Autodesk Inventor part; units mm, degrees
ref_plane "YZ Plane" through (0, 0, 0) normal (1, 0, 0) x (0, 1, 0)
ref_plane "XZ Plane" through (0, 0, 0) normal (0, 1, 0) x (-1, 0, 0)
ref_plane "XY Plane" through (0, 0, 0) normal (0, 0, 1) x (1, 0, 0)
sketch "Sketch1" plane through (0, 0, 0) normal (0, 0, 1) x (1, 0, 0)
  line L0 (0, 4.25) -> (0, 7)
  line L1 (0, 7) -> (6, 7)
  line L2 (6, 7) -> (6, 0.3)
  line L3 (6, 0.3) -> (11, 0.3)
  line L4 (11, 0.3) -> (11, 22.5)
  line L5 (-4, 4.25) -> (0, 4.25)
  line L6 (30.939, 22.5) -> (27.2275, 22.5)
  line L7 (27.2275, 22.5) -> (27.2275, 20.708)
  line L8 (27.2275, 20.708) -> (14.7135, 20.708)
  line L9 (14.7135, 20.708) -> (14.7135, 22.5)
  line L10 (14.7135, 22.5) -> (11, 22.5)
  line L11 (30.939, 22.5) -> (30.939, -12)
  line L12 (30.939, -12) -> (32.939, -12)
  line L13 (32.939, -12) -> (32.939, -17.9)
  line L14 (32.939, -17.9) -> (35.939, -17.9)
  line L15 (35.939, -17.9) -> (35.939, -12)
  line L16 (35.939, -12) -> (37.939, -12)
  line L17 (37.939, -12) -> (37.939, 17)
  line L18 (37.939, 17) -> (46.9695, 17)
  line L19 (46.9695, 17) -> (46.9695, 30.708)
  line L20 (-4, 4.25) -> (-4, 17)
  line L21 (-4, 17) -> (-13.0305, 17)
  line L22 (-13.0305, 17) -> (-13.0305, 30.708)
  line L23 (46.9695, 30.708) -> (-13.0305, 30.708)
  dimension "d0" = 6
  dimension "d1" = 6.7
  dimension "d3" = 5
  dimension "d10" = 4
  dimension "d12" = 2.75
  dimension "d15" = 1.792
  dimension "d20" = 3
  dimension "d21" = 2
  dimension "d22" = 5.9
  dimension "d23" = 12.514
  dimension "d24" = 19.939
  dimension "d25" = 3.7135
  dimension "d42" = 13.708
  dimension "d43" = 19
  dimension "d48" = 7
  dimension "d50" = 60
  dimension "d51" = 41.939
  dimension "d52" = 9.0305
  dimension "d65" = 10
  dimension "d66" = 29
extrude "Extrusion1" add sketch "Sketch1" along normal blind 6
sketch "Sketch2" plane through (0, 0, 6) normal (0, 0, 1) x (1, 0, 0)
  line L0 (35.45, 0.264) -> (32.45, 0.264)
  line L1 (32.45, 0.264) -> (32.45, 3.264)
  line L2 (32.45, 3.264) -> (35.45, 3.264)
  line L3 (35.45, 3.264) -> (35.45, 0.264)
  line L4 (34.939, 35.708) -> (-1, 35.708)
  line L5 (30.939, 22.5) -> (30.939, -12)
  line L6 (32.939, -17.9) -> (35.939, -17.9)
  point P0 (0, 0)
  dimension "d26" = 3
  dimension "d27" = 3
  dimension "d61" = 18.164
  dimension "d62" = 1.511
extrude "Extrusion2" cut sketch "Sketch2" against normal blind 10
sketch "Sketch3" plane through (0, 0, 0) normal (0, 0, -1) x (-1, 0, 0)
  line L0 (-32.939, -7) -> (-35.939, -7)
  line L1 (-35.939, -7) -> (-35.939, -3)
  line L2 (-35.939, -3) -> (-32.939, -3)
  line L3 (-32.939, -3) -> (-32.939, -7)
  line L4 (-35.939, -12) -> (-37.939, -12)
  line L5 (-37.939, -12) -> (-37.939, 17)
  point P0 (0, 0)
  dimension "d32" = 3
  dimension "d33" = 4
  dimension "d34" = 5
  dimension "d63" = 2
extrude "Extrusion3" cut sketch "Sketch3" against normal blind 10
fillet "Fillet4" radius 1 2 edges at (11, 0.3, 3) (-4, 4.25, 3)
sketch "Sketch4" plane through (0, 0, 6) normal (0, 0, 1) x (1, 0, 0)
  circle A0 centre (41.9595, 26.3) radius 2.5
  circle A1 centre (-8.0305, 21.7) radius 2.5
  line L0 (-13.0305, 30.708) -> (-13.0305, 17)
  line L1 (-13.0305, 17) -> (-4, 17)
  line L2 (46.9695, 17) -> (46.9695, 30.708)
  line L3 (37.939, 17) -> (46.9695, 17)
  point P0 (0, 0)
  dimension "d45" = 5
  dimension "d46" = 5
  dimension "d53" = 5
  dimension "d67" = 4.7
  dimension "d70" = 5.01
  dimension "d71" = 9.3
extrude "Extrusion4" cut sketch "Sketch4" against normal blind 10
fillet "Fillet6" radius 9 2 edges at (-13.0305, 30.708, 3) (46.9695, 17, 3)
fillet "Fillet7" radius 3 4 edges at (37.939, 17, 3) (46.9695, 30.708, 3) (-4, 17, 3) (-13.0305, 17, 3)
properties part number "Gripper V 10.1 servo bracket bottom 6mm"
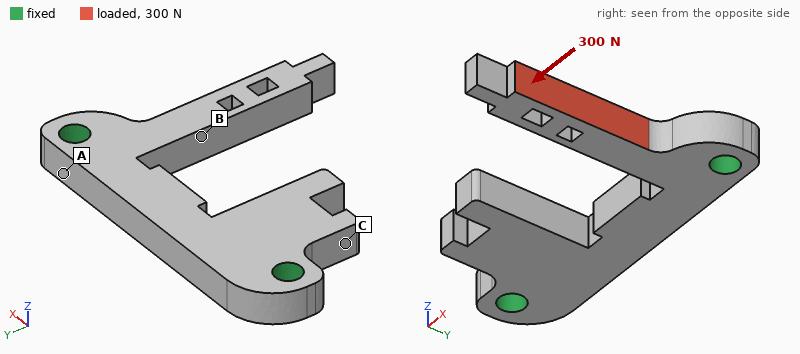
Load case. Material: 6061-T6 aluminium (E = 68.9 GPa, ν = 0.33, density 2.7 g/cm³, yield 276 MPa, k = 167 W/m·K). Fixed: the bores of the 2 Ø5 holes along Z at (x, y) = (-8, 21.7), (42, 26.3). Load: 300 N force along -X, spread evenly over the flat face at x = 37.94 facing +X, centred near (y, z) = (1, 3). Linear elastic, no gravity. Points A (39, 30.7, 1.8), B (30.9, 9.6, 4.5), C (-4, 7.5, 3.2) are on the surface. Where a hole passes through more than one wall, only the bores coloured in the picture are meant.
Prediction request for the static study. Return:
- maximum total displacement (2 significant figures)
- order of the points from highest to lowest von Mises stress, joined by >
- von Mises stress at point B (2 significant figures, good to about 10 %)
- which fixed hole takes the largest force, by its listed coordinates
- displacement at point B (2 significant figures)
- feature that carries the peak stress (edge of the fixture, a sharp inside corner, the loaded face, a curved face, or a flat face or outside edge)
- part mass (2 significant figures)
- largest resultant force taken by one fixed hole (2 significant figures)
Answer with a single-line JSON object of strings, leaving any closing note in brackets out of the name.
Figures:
{"maximum total displacement": "0.19 mm", "order of the points from highest to lowest von Mises stress, joined by >": "B > A > C", "von Mises stress at point B": "54 MPa", "which fixed hole takes the largest force, by its listed coordinates": "(42, 26.3)", "displacement at point B": "0.038 mm", "feature that carries the peak stress": "a curved face", "part mass": "17 g", "largest resultant force taken by one fixed hole": "370 N"}
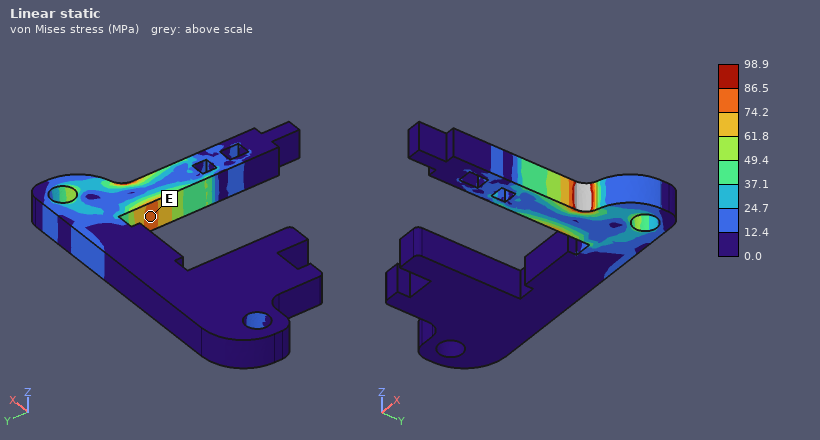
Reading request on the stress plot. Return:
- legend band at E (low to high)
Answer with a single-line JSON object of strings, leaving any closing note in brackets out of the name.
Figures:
{"legend band at E": "74.2 to 86.5 MPa"}
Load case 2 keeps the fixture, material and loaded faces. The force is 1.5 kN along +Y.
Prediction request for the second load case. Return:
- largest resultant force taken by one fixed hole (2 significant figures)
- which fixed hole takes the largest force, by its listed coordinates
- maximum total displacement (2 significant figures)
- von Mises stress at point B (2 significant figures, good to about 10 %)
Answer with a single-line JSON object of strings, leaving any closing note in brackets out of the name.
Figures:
{"largest resultant force taken by one fixed hole": "1.4 kN", "which fixed hole takes the largest force, by its listed coordinates": "(42, 26.3)", "maximum total displacement": "0.19 mm", "von Mises stress at point B": "59 MPa"}
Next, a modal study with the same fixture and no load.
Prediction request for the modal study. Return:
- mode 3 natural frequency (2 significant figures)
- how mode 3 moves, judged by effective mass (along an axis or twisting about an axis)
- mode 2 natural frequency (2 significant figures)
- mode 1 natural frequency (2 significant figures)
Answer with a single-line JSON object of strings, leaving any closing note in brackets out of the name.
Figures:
{"mode 3 natural frequency": "8700 Hz", "how mode 3 moves, judged by effective mass": "along Z", "mode 2 natural frequency": "4400 Hz", "mode 1 natural frequency": "3300 Hz"}
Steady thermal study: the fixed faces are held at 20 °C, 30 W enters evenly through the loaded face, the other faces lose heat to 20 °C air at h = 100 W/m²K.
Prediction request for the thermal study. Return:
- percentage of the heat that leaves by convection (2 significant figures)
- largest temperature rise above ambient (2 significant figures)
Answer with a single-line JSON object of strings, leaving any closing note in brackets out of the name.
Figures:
{"percentage of the heat that leaves by convection": "21 %", "largest temperature rise above ambient": "85 K"}
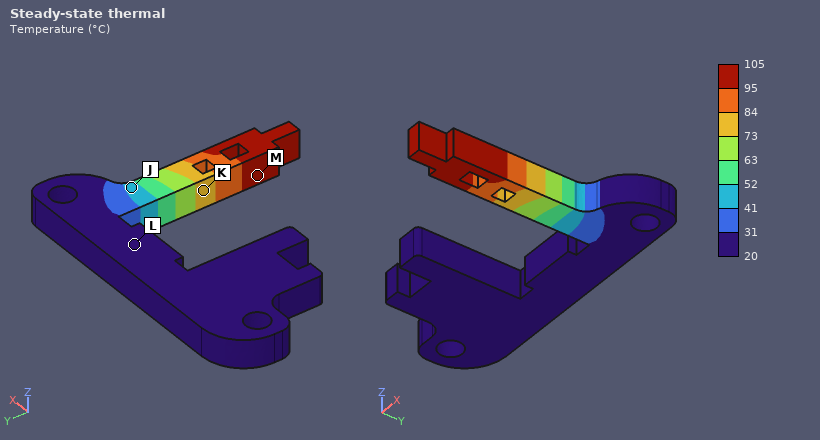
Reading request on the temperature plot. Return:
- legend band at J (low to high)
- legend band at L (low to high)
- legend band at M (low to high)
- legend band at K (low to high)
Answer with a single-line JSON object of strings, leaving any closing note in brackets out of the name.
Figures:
{"legend band at J": "41 to 52 °C", "legend band at L": "20 to 31 °C", "legend band at M": "95 to 105 °C", "legend band at K": "73 to 84 °C"}
